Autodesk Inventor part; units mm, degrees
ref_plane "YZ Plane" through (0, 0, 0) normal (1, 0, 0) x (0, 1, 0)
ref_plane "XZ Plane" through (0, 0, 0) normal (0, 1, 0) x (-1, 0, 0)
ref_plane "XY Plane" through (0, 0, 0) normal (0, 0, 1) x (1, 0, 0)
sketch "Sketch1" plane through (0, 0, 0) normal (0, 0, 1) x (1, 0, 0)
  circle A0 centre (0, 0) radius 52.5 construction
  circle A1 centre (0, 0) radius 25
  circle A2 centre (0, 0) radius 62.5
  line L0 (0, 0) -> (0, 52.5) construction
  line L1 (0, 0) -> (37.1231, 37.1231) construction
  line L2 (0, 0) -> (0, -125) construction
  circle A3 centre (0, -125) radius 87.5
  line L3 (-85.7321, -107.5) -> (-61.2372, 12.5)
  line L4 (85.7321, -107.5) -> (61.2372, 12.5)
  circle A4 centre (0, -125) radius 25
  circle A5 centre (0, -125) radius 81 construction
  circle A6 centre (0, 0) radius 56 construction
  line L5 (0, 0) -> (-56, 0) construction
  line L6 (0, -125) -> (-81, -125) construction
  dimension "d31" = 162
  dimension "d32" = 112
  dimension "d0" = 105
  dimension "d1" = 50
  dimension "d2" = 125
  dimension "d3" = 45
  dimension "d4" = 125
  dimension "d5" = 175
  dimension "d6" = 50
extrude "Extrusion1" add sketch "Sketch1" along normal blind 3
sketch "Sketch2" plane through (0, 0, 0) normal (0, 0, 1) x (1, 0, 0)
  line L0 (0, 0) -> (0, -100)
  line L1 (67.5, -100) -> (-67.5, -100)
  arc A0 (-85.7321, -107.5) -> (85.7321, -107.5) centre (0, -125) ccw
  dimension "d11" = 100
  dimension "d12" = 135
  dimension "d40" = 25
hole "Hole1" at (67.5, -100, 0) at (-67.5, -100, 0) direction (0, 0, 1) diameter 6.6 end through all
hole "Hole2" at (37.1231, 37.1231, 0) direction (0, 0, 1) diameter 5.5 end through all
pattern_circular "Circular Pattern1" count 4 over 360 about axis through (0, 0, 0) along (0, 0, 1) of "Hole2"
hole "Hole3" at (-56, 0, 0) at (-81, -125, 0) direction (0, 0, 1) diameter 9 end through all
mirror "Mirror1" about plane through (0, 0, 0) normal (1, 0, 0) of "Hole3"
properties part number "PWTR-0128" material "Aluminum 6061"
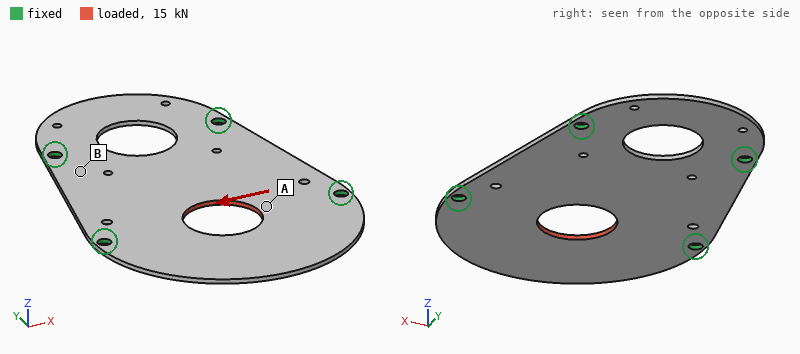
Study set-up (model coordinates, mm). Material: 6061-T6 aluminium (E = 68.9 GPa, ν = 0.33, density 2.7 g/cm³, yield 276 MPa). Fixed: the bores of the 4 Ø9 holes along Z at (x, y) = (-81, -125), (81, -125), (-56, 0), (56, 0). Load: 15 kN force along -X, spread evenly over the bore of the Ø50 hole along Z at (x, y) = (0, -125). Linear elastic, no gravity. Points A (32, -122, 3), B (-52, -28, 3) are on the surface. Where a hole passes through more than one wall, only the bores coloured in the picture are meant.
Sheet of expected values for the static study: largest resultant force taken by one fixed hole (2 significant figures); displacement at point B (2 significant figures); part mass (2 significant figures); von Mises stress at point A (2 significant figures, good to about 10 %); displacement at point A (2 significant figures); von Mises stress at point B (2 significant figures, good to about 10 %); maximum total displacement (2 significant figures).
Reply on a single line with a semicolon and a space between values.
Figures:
6.5 kN; 14 µm; 270 g; 38 MPa; 40 µm; 12 MPa; 60 µm
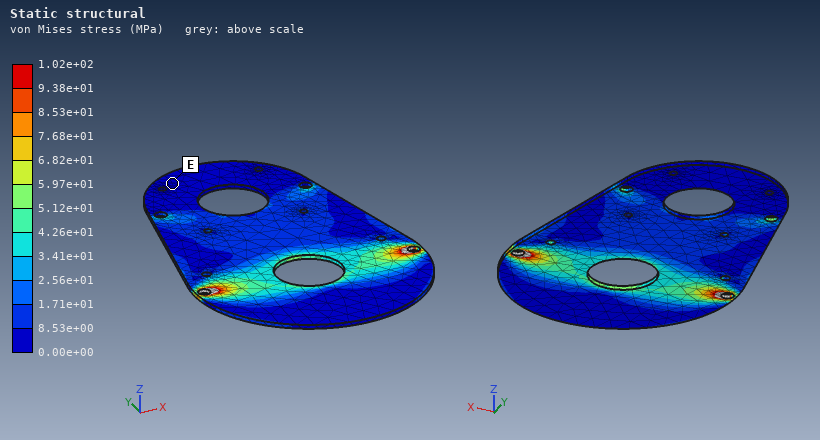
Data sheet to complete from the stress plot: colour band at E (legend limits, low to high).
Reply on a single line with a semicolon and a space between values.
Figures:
0.00e+00 to 8.53e+00 MPa
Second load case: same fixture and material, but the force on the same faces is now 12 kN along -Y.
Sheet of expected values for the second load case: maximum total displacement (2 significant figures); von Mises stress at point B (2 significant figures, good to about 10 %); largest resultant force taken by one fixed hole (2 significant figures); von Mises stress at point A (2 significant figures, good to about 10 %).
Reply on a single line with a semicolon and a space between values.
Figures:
54 µm; 21 MPa; 3.5 kN; 29 MPa
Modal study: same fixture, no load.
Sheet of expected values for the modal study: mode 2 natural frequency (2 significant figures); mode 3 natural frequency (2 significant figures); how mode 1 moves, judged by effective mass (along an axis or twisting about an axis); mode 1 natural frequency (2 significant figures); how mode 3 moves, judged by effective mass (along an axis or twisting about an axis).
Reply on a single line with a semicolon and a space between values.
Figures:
560 Hz; 620 Hz; along Z; 280 Hz; along Z
